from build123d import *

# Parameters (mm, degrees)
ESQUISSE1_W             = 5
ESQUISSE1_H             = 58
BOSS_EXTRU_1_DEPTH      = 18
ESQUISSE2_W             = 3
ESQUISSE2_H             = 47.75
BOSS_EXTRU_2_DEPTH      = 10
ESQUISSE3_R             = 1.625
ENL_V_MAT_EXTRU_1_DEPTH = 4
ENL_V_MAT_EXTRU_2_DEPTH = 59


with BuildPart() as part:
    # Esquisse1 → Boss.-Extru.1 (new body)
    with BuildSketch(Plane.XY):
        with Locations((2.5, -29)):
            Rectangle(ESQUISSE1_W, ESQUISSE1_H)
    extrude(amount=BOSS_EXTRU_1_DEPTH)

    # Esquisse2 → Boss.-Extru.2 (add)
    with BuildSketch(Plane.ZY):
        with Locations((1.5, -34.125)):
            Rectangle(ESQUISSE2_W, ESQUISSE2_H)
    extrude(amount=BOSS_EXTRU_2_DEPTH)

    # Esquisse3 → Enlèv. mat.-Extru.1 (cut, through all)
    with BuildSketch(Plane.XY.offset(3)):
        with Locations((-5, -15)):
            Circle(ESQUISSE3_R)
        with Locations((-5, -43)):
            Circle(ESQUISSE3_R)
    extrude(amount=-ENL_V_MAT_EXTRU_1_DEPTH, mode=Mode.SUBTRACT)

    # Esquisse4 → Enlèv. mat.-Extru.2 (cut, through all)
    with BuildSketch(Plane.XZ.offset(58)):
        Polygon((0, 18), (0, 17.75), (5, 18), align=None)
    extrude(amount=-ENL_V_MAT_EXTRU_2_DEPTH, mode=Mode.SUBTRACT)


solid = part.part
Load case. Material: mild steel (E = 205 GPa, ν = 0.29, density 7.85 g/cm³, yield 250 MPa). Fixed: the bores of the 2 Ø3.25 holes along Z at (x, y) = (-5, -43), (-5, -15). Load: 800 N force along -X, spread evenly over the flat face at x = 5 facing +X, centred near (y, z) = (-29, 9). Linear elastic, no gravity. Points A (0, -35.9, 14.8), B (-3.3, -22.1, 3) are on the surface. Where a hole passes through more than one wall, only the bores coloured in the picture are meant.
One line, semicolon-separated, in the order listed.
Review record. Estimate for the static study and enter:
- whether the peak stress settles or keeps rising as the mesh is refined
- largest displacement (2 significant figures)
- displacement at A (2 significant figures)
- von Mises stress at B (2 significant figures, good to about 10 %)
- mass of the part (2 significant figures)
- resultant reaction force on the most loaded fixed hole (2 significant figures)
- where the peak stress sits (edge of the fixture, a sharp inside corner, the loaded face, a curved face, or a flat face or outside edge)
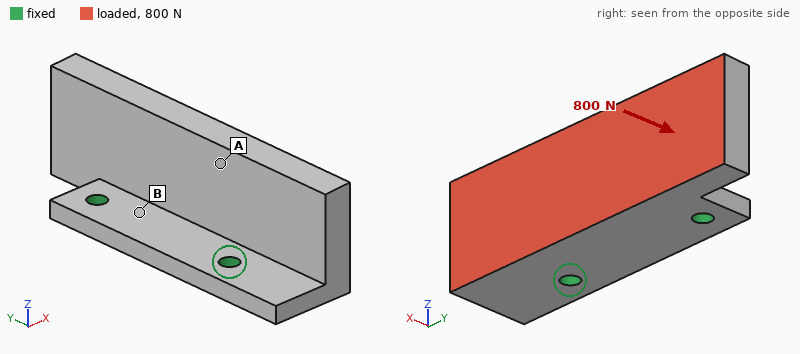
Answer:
keeps rising; 48 µm; 31 µm; 57 MPa; 52 g; 410 N; edge of the fixture
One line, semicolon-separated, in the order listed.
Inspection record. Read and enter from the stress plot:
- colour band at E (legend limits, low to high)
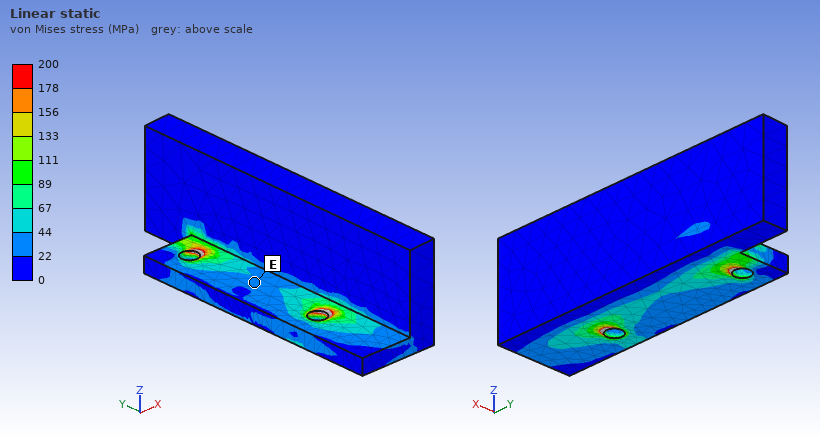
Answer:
22 to 44 MPa
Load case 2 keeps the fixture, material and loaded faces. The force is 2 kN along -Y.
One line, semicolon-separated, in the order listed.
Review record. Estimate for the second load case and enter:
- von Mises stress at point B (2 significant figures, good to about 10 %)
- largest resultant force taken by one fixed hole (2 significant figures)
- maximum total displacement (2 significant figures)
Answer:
43 MPa; 1.3 kN; 12 µm
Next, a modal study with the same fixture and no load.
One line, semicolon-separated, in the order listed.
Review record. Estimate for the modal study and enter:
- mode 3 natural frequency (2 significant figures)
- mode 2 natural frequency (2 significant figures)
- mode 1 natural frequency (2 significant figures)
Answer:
11 kHz; 6800 Hz; 3900 Hz
